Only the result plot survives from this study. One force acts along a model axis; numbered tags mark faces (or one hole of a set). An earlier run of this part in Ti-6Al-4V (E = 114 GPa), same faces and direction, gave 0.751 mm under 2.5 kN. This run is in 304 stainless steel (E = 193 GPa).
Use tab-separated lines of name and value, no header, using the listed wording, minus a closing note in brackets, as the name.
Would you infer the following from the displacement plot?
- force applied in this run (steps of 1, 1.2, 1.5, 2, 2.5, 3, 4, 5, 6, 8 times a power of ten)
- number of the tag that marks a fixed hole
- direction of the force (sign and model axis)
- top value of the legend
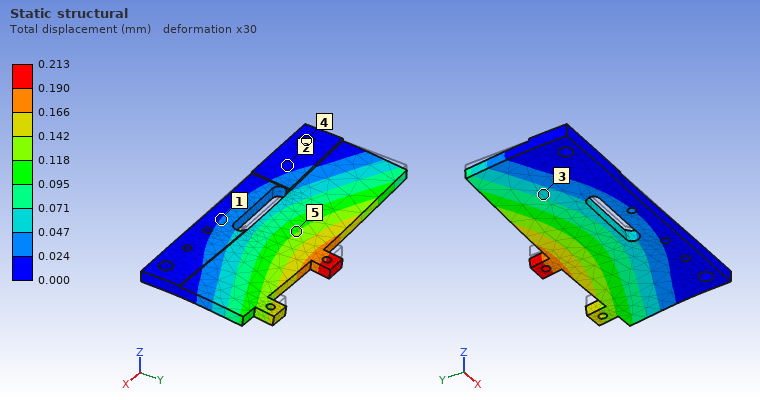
force applied in this run	1.2 kN
number of the tag that marks a fixed hole	4
direction of the force	-Z
top value of the legend	0.213 mm
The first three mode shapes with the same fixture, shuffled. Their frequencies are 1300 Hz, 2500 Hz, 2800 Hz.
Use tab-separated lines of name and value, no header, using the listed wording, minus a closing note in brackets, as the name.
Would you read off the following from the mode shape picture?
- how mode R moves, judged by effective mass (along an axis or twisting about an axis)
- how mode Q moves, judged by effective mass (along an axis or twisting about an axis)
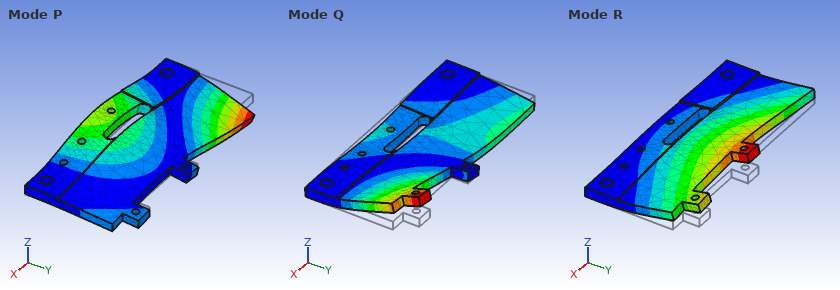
how mode R moves, judged by effective mass	along Z
how mode Q moves, judged by effective mass	twisting about Y
